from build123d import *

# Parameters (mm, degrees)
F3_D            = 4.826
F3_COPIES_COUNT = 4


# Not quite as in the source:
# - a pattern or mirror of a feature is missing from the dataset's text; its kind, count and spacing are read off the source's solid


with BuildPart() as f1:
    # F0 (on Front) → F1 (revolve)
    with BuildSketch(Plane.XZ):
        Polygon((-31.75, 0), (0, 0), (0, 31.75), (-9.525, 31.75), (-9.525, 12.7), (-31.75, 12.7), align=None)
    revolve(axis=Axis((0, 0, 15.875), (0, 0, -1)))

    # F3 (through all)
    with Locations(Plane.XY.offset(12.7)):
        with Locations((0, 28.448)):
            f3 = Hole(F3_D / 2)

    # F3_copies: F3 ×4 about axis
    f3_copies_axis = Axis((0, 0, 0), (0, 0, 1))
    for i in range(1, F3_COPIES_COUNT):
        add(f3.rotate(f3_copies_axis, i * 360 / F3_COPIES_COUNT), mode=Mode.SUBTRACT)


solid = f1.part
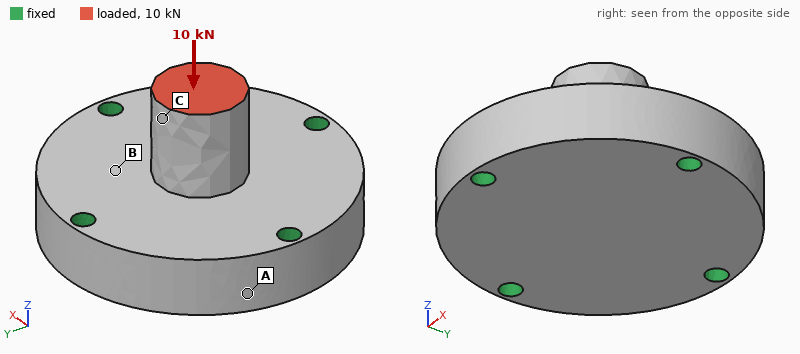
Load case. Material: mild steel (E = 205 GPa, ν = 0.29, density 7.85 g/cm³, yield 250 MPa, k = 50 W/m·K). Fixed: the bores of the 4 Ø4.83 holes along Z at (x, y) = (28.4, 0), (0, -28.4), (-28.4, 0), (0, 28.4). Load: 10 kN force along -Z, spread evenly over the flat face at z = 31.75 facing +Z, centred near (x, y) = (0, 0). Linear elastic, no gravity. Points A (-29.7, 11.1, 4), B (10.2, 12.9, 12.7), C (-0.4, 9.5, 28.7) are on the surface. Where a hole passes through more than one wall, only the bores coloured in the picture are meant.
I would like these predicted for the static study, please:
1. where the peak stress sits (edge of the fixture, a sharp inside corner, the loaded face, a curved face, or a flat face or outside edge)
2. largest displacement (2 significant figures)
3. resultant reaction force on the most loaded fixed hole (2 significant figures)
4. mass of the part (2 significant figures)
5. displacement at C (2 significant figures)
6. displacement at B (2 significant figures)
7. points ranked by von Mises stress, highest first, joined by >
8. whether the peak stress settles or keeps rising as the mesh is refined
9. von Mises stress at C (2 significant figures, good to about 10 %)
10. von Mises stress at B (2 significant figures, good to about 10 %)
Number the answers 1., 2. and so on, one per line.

1. edge of the fixture
2. 9.7 µm
3. 2.5 kN
4. 350 g
5. 9.1 µm
6. 3.8 µm
7. C > B > A
8. keeps rising
9. 35 MPa
10. 18 MPa
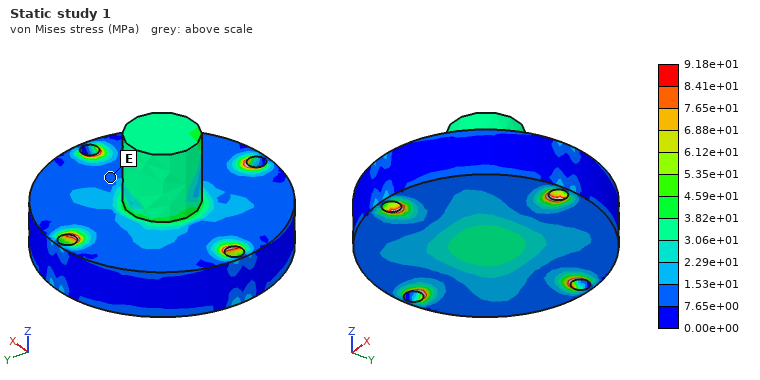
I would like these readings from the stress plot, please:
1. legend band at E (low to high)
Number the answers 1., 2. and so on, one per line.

1. 7.65e+00 to 1.53e+01 MPa
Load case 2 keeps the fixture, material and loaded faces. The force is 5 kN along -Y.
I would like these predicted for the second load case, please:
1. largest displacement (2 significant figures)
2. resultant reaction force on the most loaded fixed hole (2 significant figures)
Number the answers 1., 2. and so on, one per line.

1. 28 µm
2. 2.9 kN
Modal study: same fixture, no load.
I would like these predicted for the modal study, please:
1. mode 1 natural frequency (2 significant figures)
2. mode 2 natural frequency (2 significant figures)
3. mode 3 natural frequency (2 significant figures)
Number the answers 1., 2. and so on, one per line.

1. 17 kHz
2. 17 kHz
3. 17 kHz
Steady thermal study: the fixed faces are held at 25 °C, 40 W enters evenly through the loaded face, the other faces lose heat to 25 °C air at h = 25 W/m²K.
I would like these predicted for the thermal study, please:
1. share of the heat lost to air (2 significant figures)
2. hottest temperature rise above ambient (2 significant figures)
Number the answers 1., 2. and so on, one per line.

1. 6.5 %
2. 76 K
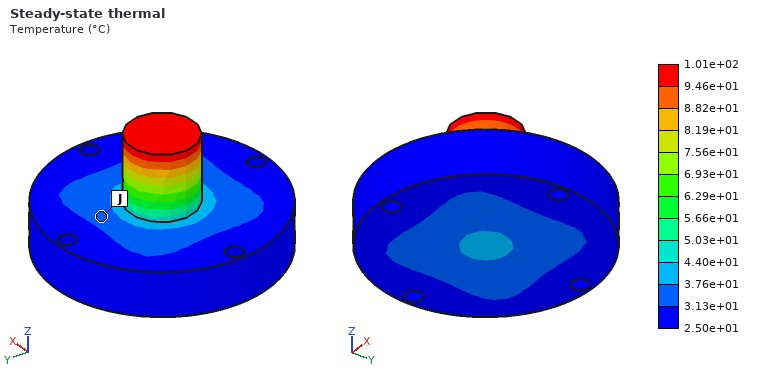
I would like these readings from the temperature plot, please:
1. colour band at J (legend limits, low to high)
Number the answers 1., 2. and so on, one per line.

1. 3.13e+01 to 3.76e+01 °C
